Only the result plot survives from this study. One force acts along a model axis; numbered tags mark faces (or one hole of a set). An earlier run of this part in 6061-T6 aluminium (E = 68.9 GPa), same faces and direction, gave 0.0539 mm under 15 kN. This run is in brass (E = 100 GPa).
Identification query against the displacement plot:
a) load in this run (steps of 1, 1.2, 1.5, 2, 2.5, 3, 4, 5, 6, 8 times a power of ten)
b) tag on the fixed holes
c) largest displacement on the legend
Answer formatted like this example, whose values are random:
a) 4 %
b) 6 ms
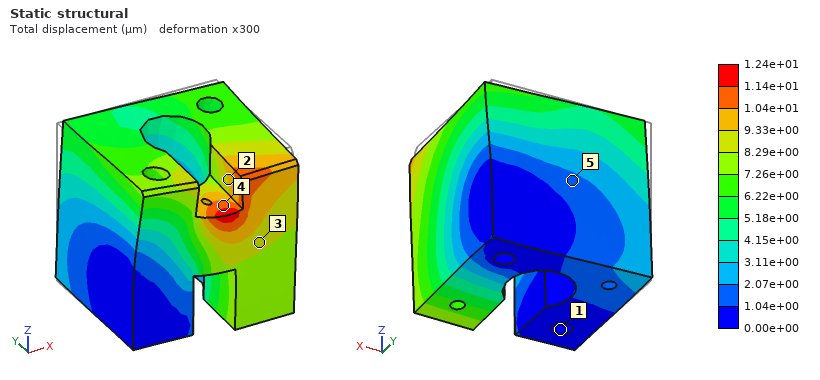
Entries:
a) 5 kN
b) 1
c) 1.24e+01 µm
